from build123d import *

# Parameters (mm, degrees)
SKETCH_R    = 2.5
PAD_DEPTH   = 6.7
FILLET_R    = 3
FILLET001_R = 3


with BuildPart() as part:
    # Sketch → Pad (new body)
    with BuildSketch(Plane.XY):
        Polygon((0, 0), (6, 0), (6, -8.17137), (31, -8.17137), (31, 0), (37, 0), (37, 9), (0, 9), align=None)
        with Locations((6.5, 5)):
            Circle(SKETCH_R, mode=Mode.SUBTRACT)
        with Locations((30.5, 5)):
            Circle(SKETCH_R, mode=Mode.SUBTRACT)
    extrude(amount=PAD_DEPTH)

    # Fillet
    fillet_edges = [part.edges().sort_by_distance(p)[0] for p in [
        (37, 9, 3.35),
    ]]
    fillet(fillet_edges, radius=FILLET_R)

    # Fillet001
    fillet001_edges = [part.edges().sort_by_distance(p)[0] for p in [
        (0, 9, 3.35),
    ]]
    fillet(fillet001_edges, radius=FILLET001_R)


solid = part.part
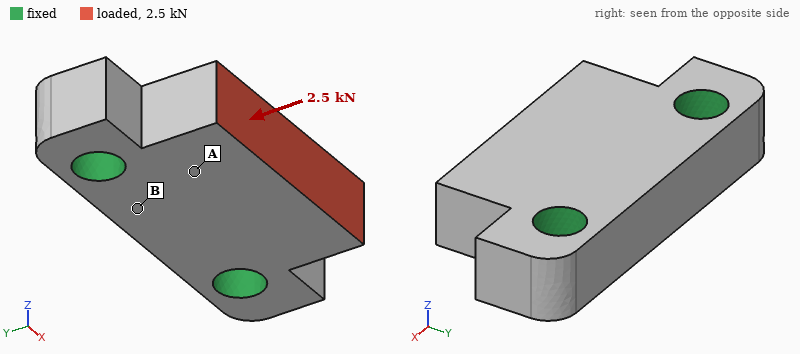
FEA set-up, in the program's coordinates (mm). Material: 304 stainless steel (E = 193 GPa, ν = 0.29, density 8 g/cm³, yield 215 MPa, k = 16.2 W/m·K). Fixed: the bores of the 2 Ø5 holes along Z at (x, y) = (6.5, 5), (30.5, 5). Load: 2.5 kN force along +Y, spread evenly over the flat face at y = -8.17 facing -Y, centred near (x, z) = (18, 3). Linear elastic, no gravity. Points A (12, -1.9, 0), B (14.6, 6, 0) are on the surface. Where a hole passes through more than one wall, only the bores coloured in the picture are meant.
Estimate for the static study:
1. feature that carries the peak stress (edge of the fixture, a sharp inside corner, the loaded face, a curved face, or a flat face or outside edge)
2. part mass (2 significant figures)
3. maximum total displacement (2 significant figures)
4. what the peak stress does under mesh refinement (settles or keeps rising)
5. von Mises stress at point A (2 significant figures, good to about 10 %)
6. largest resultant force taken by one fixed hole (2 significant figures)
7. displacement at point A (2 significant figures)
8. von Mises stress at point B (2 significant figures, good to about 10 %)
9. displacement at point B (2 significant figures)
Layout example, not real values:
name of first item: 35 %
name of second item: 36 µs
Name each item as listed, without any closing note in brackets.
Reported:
feature that carries the peak stress: edge of the fixture
part mass: 26 g
maximum total displacement: 1.6 µm
what the peak stress does under mesh refinement: keeps rising
von Mises stress at point A: 17 MPa
largest resultant force taken by one fixed hole: 1.3 kN
displacement at point A: 0.99 µm
von Mises stress at point B: 6.7 MPa
displacement at point B: 0.95 µm
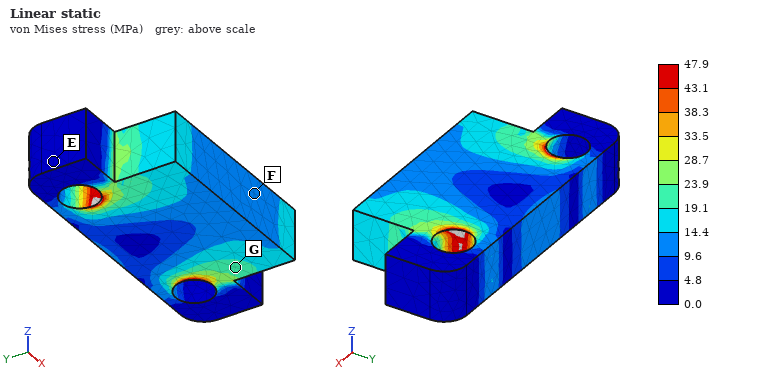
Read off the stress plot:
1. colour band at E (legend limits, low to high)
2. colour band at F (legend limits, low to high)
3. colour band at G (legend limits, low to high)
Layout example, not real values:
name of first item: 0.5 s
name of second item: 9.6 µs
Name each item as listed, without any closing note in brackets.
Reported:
colour band at E: 0.0 to 4.8 MPa
colour band at F: 9.6 to 14.4 MPa
colour band at G: 19.1 to 23.9 MPa
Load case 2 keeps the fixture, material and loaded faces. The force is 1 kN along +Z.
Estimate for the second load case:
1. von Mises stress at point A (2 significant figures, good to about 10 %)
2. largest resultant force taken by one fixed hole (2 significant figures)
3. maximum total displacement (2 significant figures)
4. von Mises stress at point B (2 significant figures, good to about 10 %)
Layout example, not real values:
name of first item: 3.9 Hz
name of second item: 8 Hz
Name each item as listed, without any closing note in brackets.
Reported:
von Mises stress at point A: 32 MPa
largest resultant force taken by one fixed hole: 500 N
maximum total displacement: 9.5 µm
von Mises stress at point B: 18 MPa
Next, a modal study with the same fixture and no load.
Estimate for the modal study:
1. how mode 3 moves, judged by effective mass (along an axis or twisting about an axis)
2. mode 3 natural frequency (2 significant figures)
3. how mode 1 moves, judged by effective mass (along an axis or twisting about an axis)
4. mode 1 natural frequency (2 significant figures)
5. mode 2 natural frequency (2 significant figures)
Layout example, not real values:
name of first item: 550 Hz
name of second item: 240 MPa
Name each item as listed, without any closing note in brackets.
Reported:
how mode 3 moves, judged by effective mass: along Z
mode 3 natural frequency: 52 kHz
how mode 1 moves, judged by effective mass: along Z
mode 1 natural frequency: 24 kHz
mode 2 natural frequency: 42 kHz
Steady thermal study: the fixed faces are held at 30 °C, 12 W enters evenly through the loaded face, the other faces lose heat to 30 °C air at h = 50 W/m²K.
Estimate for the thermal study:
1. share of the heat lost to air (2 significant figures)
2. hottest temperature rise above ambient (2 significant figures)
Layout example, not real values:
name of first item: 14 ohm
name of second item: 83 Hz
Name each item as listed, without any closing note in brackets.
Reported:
share of the heat lost to air: 11 %
hottest temperature rise above ambient: 59 K
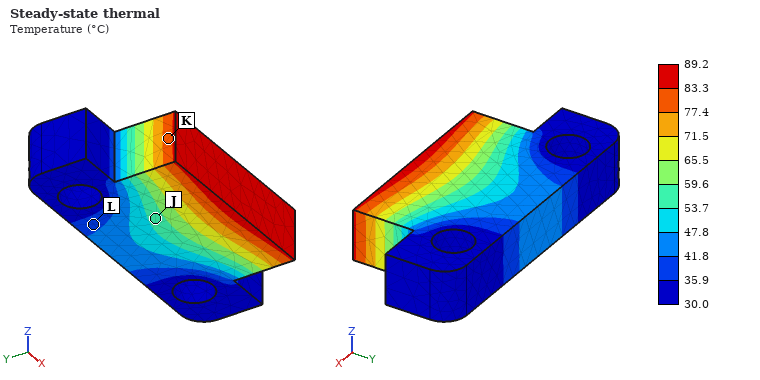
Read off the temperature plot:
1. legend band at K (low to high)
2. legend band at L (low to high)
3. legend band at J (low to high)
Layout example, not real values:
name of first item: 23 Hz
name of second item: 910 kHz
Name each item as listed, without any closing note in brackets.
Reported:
legend band at K: 77.4 to 83.3 °C
legend band at L: 35.9 to 41.8 °C
legend band at J: 53.7 to 59.6 °C
